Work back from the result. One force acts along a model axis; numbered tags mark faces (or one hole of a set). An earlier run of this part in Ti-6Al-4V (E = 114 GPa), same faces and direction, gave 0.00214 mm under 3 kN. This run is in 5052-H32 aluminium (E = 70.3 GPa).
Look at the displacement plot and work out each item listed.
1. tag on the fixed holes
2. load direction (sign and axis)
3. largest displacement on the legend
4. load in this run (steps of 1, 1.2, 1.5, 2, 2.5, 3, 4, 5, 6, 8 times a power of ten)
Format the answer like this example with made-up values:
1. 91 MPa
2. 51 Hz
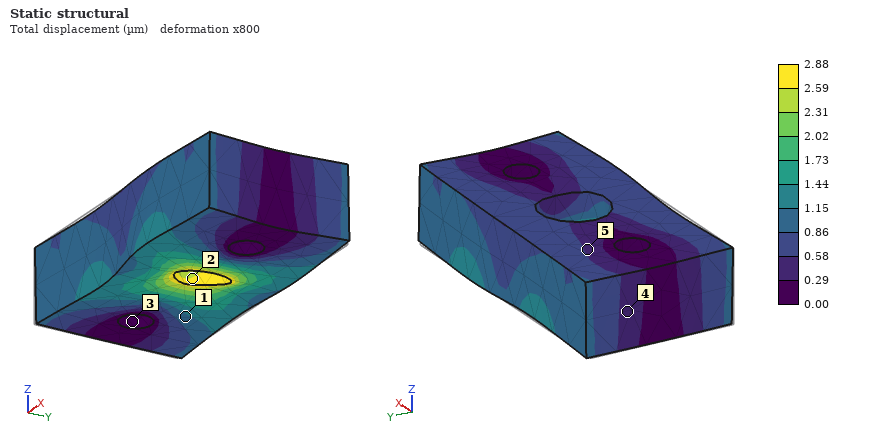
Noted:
1. 3
2. +X
3. 2.88 µm
4. 2.5 kN
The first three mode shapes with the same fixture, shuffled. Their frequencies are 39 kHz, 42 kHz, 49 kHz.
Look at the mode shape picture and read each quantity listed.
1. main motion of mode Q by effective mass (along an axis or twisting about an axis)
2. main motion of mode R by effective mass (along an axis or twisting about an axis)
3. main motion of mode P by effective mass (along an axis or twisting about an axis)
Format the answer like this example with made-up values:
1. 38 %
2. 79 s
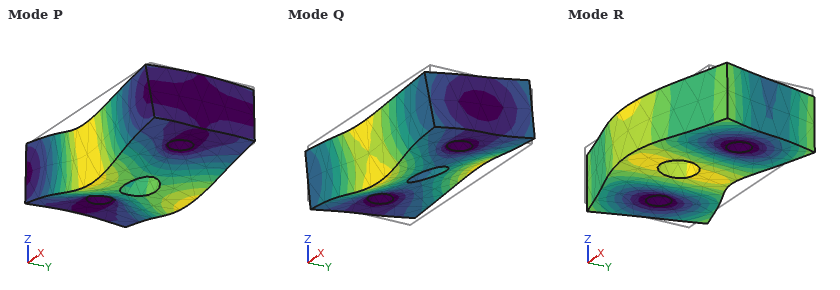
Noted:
1. twisting about X
2. along Y
3. along Z
